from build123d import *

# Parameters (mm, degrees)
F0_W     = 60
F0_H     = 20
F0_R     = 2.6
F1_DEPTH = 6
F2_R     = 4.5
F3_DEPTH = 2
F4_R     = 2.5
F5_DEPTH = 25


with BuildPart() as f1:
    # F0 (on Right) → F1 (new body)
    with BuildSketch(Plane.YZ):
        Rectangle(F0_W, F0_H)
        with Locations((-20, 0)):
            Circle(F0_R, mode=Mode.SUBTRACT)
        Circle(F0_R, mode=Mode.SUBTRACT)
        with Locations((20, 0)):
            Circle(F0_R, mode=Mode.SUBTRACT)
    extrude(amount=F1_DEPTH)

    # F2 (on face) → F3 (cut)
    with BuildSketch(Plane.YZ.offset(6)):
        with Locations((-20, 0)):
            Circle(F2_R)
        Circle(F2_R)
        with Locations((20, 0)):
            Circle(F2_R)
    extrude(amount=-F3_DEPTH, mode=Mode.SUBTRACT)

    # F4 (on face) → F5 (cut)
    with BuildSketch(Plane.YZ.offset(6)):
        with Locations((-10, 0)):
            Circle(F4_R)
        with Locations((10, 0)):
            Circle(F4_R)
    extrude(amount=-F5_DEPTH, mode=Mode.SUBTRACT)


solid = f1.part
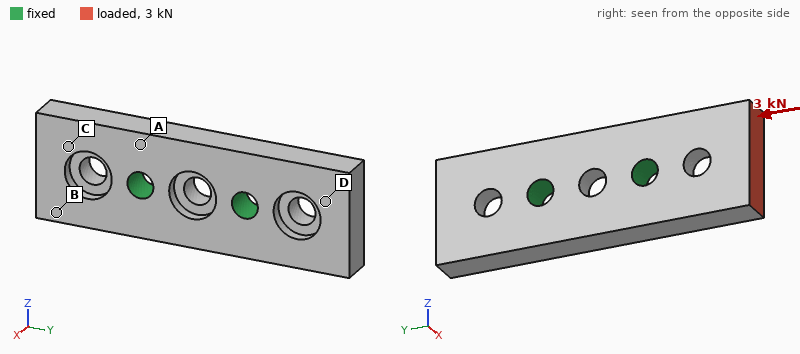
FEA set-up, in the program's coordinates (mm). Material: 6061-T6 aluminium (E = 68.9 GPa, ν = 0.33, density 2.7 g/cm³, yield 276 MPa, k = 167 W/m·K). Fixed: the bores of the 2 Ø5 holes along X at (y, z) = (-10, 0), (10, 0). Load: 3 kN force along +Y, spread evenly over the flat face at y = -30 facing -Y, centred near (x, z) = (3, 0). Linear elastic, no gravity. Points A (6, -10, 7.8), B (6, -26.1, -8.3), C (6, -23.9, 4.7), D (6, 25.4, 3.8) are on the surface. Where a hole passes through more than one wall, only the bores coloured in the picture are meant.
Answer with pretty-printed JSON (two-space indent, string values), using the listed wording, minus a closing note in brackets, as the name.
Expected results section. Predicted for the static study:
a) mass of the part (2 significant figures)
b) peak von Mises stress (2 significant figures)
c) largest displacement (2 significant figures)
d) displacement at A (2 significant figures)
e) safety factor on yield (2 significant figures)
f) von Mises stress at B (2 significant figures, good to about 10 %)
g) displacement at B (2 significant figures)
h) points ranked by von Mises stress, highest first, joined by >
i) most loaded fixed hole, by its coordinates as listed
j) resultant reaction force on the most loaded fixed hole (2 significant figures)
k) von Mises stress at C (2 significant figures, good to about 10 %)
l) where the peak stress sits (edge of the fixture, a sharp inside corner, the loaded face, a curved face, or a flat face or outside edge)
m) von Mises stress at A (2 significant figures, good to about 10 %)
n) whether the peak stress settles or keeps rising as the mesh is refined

{
  "mass of the part": "17 g",
  "peak von Mises stress": "120 MPa",
  "largest displacement": "16 µm",
  "displacement at A": "3.0 µm",
  "safety factor on yield": "2.2",
  "von Mises stress at B": "30 MPa",
  "displacement at B": "11 µm",
  "points ranked by von Mises stress, highest first, joined by >": "C > B > A > D",
  "most loaded fixed hole, by its coordinates as listed": "(-10, 0)",
  "resultant reaction force on the most loaded fixed hole": "2.5 kN",
  "von Mises stress at C": "46 MPa",
  "where the peak stress sits": "a curved face",
  "von Mises stress at A": "21 MPa",
  "whether the peak stress settles or keeps rising as the mesh is refined": "settles"
}
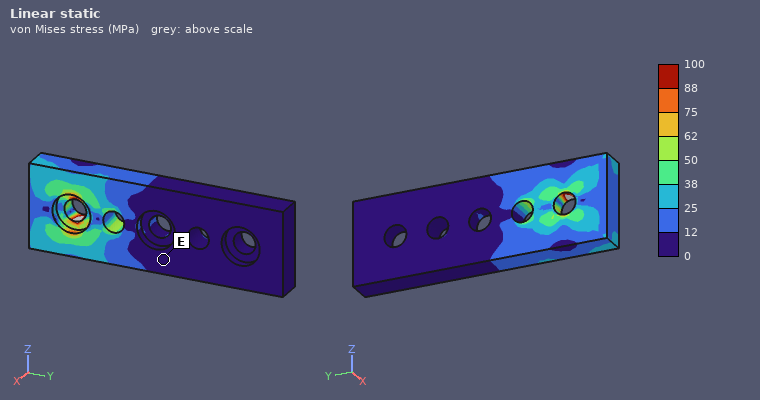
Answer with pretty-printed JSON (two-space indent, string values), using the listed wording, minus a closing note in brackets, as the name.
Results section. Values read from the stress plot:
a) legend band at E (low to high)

{
  "legend band at E": "0 to 12 MPa"
}
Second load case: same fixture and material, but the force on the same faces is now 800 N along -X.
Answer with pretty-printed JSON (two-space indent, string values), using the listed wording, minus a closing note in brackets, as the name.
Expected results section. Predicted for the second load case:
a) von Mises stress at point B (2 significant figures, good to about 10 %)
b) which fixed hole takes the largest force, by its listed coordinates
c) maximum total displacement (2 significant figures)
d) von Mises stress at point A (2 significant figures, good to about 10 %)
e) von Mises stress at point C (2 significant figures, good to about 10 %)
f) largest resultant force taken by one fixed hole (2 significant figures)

{
  "von Mises stress at point B": "35 MPa",
  "which fixed hole takes the largest force, by its listed coordinates": "(-10, 0)",
  "maximum total displacement": "0.12 mm",
  "von Mises stress at point A": "64 MPa",
  "von Mises stress at point C": "58 MPa",
  "largest resultant force taken by one fixed hole": "980 N"
}
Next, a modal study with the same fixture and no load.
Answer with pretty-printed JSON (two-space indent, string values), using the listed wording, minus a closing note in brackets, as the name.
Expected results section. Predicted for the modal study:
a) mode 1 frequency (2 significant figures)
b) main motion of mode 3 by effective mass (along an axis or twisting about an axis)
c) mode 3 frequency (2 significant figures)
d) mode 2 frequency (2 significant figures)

{
  "mode 1 frequency": "11 kHz",
  "main motion of mode 3 by effective mass": "twisting about X",
  "mode 3 frequency": "18 kHz",
  "mode 2 frequency": "11 kHz"
}
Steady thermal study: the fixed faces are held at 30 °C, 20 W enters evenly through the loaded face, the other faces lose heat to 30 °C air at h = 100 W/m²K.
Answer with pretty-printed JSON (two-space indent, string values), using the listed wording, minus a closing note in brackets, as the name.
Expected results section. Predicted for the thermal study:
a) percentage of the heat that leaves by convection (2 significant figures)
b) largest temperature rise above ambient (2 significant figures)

{
  "percentage of the heat that leaves by convection": "7.0 %",
  "largest temperature rise above ambient": "23 K"
}
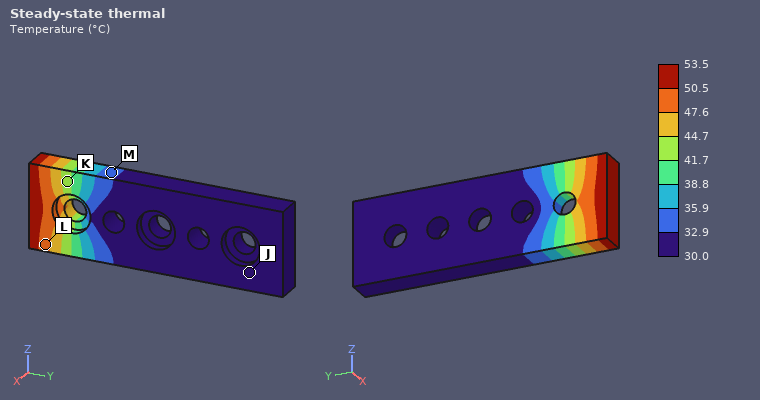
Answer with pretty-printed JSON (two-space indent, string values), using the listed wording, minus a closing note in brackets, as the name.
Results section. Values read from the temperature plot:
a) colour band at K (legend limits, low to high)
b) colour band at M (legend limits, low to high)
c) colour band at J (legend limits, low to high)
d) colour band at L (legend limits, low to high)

{
  "colour band at K": "41.7 to 44.7 °C",
  "colour band at M": "32.9 to 35.9 °C",
  "colour band at J": "30.0 to 32.9 °C",
  "colour band at L": "47.6 to 50.5 °C"
}
